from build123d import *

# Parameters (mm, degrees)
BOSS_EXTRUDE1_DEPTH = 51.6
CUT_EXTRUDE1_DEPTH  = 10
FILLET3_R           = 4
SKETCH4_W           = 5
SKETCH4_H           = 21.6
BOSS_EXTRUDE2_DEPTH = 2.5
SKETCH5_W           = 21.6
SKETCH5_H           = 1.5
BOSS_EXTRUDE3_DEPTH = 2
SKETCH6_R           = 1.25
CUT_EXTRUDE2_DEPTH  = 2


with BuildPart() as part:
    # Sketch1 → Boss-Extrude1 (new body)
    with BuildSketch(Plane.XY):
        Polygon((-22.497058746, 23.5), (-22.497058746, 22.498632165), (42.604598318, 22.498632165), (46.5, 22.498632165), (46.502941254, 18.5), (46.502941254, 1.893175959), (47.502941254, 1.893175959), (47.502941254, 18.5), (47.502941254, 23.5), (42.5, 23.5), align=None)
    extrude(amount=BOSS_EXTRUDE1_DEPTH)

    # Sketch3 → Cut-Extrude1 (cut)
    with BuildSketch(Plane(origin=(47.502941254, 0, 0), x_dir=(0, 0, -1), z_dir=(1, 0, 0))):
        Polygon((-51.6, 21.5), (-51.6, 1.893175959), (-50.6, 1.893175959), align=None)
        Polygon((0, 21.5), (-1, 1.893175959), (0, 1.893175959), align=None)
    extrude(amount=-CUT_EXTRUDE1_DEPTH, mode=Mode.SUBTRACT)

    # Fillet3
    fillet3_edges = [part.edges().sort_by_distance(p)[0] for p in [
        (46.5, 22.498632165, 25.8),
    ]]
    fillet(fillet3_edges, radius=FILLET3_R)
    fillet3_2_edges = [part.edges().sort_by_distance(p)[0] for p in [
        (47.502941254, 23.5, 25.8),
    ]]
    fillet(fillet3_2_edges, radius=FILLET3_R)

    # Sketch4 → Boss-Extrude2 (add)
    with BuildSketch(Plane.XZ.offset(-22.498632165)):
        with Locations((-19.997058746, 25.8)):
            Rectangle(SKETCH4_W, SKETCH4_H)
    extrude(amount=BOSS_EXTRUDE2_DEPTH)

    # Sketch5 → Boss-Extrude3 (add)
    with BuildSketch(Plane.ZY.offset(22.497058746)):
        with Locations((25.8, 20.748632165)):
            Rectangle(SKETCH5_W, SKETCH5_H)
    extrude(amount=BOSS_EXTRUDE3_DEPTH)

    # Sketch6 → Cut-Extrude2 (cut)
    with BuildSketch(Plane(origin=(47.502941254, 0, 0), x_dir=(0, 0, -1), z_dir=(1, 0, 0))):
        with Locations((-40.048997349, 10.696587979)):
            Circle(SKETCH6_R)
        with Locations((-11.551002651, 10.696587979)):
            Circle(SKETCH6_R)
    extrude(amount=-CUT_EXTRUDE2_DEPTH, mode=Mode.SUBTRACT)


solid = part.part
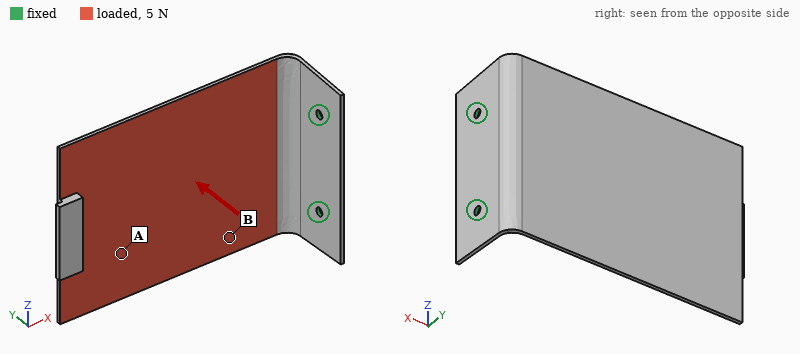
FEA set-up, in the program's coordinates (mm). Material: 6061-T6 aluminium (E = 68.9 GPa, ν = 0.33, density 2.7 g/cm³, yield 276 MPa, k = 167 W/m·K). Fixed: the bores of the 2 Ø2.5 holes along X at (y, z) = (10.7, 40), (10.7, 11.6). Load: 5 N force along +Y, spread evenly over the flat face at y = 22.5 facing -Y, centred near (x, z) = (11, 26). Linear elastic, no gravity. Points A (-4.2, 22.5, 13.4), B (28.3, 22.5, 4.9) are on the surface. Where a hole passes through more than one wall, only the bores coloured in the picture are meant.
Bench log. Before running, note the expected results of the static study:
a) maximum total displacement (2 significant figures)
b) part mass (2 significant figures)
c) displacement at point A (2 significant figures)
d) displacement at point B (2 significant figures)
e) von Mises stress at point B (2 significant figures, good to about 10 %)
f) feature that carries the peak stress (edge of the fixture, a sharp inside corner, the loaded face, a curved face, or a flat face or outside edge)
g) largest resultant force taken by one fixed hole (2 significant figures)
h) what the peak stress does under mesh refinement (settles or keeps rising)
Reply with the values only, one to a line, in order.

1.1 mm
13 g
0.70 mm
0.18 mm
11 MPa
edge of the fixture
2.7 N
keeps rising
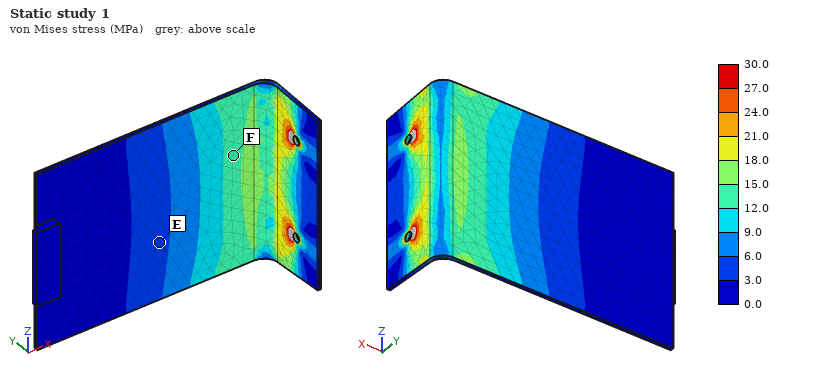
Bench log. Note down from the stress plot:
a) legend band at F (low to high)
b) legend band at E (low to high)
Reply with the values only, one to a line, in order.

12.0 to 15.0 MPa
3.0 to 6.0 MPa
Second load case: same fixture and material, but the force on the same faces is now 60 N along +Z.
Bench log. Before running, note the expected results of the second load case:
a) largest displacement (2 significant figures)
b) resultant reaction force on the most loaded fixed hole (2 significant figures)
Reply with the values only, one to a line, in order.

0.93 mm
78 N
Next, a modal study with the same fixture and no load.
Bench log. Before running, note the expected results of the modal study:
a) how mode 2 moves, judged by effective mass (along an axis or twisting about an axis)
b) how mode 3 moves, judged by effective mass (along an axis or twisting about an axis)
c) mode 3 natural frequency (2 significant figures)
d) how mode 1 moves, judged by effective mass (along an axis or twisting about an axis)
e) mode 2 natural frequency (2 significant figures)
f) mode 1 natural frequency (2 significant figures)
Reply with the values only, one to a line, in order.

along Z
along Z
610 Hz
along Y
410 Hz
120 Hz
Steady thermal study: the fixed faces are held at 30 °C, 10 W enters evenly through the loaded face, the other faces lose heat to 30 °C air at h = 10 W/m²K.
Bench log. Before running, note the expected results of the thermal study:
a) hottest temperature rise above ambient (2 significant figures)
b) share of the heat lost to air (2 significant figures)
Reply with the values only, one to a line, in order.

48 K
18 %
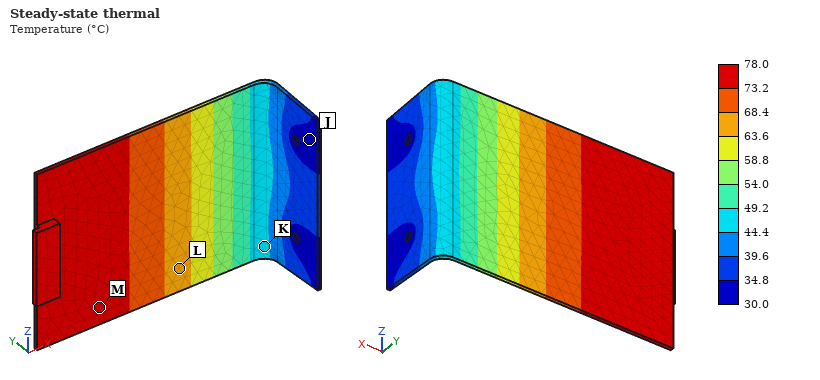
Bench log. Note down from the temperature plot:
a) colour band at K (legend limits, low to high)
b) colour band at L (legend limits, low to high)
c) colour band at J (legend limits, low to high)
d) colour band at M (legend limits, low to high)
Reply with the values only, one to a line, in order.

44.4 to 49.2 °C
63.6 to 68.4 °C
30.0 to 34.8 °C
73.2 to 78.0 °C
